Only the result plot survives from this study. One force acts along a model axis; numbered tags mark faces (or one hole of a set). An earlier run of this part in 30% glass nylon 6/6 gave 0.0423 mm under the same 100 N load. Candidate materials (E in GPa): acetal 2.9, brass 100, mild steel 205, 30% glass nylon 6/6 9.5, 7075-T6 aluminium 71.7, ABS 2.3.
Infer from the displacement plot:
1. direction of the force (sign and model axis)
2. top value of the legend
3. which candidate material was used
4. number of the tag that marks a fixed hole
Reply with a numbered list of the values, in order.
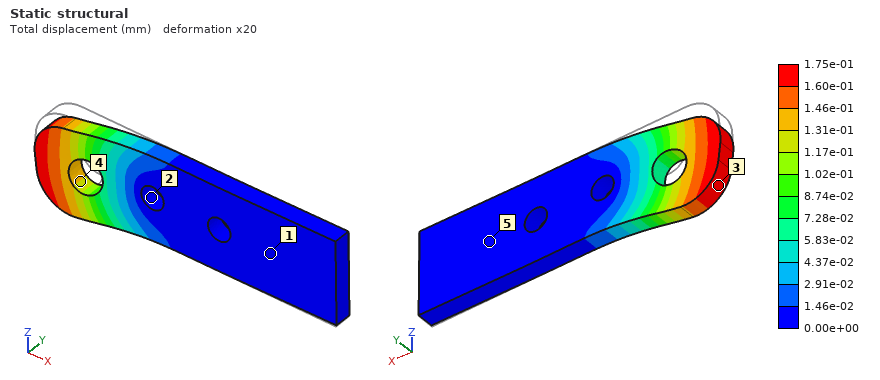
1. -Z
2. 1.75e-01 mm
3. ABS
4. 2
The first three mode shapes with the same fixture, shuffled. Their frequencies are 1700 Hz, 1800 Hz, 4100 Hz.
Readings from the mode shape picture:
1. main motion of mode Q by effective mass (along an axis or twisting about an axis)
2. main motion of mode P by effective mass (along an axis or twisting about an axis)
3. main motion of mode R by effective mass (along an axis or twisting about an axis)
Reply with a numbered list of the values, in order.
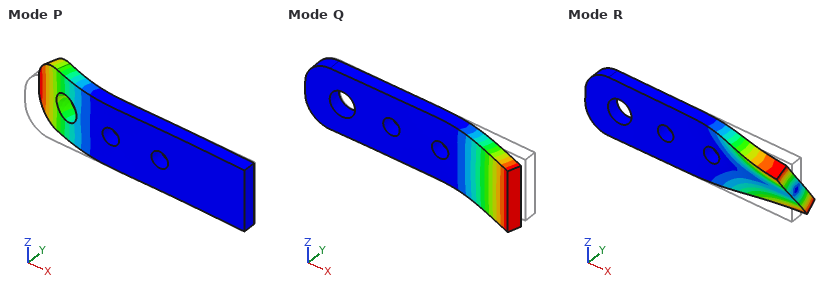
1. along Y
2. along Y
3. twisting about X
